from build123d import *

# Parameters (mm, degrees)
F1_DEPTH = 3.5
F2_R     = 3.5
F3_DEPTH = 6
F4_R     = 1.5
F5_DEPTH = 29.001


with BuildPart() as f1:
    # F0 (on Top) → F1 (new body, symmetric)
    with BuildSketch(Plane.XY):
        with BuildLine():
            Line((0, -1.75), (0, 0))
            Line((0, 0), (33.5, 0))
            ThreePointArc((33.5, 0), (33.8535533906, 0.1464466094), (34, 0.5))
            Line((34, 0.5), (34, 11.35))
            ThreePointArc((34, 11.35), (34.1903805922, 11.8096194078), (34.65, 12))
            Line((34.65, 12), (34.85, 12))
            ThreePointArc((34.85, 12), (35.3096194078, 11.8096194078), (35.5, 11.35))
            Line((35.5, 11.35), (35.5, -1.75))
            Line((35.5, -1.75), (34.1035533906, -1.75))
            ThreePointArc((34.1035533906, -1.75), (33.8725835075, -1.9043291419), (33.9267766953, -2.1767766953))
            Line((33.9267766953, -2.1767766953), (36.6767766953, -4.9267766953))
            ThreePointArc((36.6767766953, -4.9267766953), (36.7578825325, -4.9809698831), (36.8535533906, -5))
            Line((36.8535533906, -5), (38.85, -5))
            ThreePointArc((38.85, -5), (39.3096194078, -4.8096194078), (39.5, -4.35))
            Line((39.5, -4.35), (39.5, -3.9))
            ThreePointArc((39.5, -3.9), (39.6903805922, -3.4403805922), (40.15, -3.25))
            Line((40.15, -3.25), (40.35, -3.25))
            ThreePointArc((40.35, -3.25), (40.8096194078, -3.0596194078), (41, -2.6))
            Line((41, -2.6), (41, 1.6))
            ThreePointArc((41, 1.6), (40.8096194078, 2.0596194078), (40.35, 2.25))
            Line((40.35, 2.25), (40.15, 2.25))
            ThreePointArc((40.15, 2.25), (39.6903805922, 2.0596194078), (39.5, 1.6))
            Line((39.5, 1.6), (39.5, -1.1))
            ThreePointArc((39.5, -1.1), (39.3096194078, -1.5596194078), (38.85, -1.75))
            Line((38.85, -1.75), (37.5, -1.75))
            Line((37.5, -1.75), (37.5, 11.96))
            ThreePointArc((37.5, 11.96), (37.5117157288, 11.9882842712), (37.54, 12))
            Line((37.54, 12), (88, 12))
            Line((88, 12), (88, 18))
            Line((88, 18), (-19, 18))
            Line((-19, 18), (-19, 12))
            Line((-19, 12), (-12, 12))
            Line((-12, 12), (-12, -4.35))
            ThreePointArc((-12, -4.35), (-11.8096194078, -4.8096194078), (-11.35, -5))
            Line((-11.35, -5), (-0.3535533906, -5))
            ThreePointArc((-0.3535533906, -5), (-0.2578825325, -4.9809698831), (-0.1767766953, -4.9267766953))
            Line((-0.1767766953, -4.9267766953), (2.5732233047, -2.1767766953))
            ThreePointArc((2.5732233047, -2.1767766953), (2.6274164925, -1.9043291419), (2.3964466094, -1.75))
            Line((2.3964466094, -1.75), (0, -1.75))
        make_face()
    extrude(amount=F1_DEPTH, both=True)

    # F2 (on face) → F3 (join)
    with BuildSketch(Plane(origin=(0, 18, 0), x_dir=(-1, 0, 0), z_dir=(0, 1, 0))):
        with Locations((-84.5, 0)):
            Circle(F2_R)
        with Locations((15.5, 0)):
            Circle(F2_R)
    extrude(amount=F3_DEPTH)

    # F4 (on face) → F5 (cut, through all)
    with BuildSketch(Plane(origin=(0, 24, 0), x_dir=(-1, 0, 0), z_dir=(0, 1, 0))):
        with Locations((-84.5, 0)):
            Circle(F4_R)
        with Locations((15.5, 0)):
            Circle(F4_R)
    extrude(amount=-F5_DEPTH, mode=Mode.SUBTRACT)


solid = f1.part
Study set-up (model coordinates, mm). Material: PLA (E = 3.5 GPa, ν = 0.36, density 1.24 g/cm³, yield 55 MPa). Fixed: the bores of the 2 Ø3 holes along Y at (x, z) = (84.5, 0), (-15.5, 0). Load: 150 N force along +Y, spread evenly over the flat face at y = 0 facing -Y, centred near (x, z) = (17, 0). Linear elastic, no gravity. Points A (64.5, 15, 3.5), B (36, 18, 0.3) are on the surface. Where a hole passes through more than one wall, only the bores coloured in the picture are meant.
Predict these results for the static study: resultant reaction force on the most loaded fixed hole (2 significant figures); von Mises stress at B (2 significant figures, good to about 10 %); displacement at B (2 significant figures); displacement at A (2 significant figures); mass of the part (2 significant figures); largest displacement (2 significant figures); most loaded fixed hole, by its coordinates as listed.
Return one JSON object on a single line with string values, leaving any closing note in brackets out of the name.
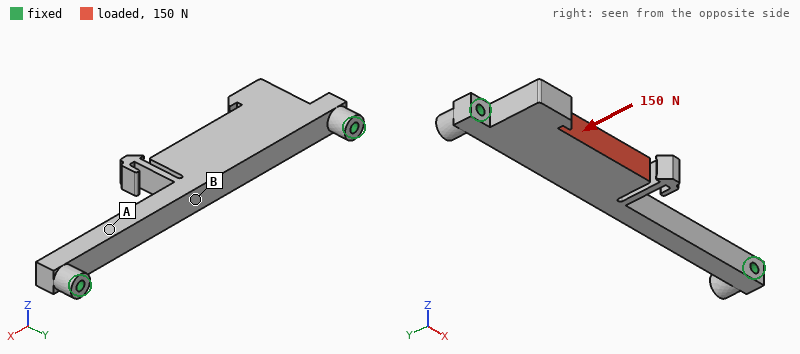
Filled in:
{"resultant reaction force on the most loaded fixed hole": "110 N", "von Mises stress at B": "21 MPa", "displacement at B": "0.76 mm", "displacement at A": "0.28 mm", "mass of the part": "12 g", "largest displacement": "0.80 mm", "most loaded fixed hole, by its coordinates as listed": "(-15.5, 0)"}
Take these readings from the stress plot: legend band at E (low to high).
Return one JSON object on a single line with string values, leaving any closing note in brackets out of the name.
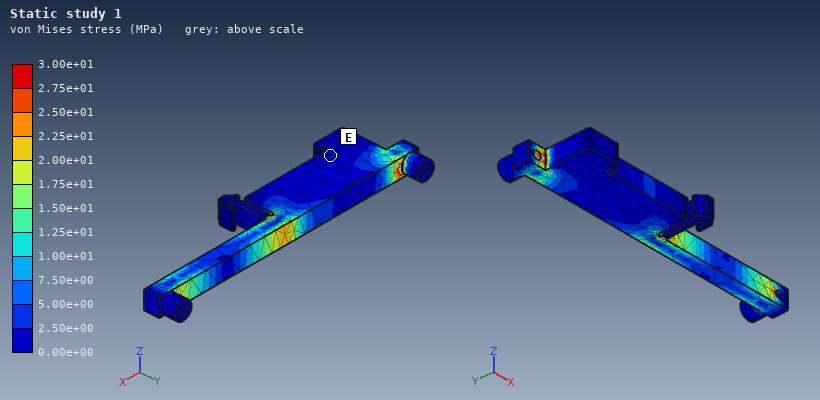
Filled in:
{"legend band at E": "0.00e+00 to 2.50e+00 MPa"}
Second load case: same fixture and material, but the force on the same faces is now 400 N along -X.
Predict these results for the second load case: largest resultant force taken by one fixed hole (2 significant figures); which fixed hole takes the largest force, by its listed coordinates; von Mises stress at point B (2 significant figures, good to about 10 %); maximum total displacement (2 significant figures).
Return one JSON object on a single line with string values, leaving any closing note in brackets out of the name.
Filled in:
{"largest resultant force taken by one fixed hole": "310 N", "which fixed hole takes the largest force, by its listed coordinates": "(-15.5, 0)", "von Mises stress at point B": "29 MPa", "maximum total displacement": "1.1 mm"}
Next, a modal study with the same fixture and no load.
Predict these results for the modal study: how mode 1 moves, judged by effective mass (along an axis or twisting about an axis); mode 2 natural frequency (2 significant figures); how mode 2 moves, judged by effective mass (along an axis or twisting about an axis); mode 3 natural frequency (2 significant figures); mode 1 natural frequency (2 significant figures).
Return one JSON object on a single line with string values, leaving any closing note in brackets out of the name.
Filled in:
{"how mode 1 moves, judged by effective mass": "along Z", "mode 2 natural frequency": "850 Hz", "how mode 2 moves, judged by effective mass": "along Y", "mode 3 natural frequency": "1200 Hz", "mode 1 natural frequency": "800 Hz"}
